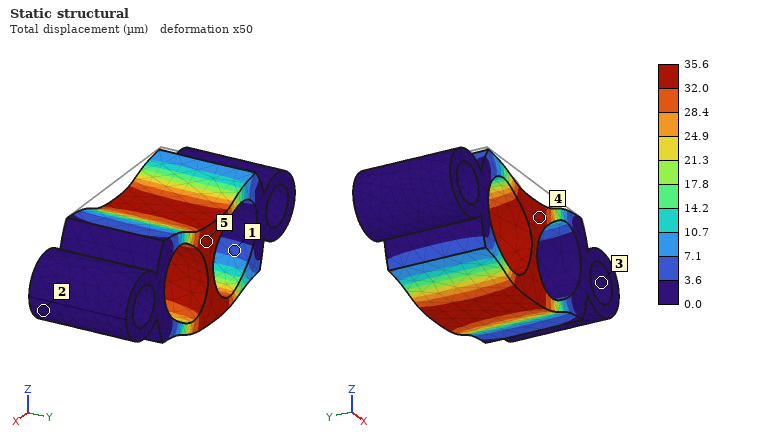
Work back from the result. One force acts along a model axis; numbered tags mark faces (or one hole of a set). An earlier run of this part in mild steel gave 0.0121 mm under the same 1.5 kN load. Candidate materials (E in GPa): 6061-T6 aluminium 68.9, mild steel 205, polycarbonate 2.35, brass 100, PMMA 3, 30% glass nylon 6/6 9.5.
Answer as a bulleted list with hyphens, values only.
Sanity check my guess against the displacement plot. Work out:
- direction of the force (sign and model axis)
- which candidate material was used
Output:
- -Z
- 6061-T6 aluminium
